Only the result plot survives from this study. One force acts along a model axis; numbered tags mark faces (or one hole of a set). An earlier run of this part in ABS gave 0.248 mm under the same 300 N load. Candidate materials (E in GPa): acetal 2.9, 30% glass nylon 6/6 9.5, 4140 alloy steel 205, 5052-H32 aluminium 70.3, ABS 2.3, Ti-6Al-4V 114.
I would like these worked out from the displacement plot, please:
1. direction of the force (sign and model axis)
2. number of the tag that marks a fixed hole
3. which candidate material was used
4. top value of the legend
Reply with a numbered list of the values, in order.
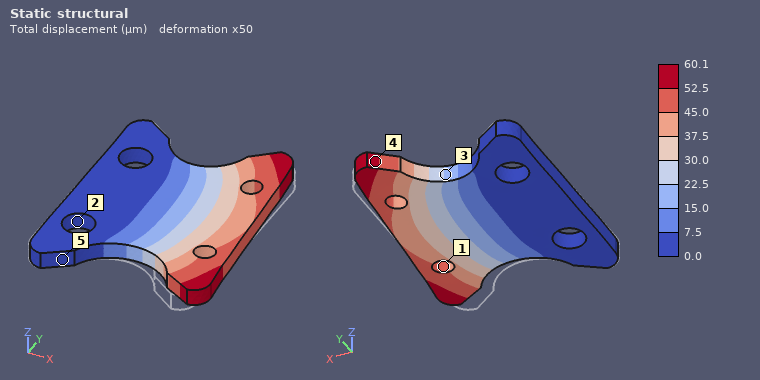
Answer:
1. +Y
2. 2
3. 30% glass nylon 6/6
4. 60.1 µm
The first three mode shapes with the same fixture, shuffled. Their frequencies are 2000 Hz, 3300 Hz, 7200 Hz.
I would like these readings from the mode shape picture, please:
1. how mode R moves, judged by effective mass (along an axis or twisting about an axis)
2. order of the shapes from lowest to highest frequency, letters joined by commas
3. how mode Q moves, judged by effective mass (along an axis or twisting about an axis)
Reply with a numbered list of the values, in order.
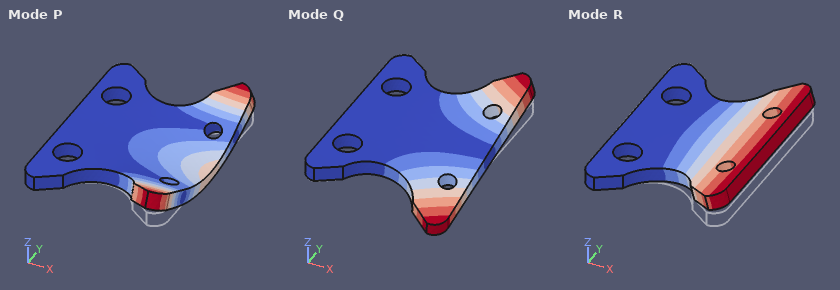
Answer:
1. along Z
2. R, Q, P
3. twisting about X
